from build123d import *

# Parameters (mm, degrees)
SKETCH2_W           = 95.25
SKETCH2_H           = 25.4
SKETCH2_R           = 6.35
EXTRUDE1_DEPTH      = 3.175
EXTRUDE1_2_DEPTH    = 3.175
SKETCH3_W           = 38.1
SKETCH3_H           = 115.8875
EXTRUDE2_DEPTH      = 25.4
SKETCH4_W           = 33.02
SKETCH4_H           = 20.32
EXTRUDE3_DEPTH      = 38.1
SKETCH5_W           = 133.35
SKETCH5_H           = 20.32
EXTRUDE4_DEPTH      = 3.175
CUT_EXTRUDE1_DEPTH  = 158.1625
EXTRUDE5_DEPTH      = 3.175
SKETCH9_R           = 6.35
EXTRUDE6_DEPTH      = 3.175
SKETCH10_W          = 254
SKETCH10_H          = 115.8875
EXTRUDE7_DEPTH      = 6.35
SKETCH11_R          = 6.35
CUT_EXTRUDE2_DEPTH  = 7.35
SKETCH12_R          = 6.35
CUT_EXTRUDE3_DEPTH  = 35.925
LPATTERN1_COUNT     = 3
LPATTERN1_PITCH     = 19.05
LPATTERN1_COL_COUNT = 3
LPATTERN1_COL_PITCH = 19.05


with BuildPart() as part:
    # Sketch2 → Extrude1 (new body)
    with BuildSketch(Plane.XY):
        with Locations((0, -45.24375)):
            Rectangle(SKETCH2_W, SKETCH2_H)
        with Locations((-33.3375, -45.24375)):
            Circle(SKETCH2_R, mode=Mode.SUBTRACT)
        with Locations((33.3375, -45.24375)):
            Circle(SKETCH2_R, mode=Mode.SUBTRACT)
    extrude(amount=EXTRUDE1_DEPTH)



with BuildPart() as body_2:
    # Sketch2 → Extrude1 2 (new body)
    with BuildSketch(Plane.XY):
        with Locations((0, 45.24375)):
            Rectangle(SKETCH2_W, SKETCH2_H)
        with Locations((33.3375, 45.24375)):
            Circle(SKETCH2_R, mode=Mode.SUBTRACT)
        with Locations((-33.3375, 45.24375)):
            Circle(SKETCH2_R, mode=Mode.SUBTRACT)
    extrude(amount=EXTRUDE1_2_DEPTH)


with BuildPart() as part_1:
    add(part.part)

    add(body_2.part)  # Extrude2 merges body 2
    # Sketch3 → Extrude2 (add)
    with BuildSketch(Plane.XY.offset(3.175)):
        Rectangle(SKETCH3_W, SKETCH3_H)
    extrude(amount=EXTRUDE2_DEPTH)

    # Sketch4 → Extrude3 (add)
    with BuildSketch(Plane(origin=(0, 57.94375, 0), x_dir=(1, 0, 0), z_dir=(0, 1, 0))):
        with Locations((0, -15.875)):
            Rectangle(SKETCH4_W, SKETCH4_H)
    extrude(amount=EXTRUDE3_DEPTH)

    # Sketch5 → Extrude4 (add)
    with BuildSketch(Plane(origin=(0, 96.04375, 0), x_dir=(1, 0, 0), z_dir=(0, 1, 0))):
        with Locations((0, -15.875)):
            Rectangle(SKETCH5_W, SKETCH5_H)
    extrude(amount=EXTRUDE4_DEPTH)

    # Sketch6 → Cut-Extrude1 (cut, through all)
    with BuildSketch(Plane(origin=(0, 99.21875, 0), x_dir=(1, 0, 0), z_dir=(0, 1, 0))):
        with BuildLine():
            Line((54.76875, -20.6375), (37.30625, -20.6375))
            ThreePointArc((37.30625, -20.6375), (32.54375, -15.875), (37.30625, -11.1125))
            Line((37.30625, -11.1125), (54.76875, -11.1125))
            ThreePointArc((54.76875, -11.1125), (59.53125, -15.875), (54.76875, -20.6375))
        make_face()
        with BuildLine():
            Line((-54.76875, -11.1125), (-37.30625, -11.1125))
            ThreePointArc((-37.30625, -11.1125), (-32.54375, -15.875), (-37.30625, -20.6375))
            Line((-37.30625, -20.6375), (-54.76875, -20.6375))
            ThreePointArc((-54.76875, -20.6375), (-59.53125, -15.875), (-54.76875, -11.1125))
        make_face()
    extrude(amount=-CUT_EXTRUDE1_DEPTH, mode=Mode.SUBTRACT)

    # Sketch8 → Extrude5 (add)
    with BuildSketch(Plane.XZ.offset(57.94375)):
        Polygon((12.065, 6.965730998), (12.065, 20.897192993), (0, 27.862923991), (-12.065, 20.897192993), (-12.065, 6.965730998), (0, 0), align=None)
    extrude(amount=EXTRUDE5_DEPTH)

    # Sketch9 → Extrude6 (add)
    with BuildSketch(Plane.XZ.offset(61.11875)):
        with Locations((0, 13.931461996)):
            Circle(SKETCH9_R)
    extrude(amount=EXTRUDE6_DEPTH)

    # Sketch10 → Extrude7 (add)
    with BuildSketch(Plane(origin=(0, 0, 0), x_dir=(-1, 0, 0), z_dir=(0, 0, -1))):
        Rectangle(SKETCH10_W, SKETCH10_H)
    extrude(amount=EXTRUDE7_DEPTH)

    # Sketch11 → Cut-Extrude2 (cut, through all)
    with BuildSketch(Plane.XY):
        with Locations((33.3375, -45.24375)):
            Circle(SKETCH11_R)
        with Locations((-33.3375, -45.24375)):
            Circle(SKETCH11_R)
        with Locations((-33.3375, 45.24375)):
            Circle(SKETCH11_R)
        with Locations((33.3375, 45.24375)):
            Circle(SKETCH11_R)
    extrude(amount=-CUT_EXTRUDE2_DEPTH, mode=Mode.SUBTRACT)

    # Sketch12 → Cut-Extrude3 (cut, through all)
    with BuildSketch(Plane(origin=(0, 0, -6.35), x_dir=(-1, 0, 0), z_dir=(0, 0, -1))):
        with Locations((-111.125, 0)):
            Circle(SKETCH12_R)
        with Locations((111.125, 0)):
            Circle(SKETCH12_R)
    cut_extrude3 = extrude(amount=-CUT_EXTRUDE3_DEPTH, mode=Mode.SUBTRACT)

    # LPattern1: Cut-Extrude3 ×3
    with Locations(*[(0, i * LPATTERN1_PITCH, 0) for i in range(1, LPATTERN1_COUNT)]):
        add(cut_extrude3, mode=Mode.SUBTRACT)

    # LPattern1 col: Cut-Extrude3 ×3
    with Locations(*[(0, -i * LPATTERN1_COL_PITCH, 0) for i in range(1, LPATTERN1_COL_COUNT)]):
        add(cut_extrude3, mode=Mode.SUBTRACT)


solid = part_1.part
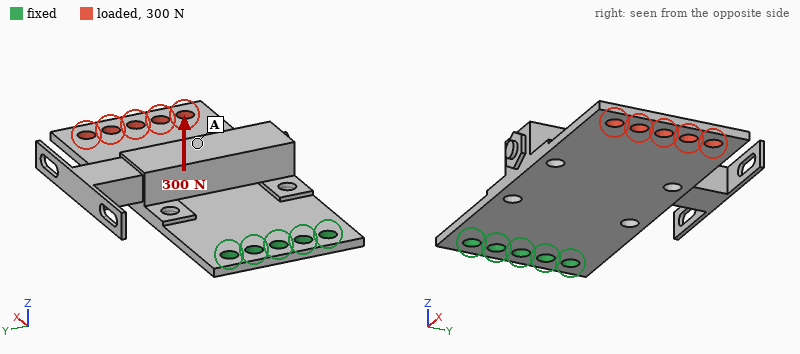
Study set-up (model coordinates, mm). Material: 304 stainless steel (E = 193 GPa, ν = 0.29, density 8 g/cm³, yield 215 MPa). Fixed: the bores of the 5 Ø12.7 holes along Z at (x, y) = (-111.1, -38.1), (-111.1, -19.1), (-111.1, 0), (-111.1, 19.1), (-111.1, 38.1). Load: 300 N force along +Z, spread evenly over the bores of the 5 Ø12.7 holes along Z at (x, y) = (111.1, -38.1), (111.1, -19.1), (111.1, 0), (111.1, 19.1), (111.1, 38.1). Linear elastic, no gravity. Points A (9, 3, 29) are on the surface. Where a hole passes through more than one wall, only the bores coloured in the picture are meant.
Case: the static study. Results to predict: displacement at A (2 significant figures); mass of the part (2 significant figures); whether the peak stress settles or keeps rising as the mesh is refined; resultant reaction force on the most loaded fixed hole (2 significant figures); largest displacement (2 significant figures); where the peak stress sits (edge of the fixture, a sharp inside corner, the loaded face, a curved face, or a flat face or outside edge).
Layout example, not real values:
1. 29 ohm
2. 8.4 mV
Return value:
1. 0.71 mm
2. 2.7 kg
3. keeps rising
4. 160 N
5. 1.8 mm
6. edge of the fixture
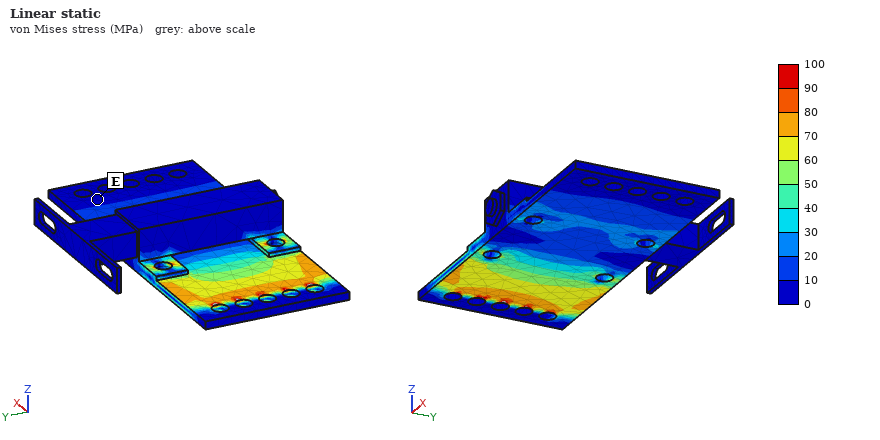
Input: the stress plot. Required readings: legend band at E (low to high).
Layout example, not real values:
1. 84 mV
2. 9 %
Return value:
1. 0 to 10 MPa
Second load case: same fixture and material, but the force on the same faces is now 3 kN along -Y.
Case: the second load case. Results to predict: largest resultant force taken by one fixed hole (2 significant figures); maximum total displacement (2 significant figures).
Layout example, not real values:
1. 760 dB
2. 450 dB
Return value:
1. 7.0 kN
2. 0.10 mm
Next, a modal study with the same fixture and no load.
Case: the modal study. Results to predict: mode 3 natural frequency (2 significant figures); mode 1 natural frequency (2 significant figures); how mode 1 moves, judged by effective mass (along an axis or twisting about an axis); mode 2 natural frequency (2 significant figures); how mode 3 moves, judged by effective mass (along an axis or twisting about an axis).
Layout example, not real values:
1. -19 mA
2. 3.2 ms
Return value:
1. 550 Hz
2. 88 Hz
3. along Z
4. 330 Hz
5. along Z
